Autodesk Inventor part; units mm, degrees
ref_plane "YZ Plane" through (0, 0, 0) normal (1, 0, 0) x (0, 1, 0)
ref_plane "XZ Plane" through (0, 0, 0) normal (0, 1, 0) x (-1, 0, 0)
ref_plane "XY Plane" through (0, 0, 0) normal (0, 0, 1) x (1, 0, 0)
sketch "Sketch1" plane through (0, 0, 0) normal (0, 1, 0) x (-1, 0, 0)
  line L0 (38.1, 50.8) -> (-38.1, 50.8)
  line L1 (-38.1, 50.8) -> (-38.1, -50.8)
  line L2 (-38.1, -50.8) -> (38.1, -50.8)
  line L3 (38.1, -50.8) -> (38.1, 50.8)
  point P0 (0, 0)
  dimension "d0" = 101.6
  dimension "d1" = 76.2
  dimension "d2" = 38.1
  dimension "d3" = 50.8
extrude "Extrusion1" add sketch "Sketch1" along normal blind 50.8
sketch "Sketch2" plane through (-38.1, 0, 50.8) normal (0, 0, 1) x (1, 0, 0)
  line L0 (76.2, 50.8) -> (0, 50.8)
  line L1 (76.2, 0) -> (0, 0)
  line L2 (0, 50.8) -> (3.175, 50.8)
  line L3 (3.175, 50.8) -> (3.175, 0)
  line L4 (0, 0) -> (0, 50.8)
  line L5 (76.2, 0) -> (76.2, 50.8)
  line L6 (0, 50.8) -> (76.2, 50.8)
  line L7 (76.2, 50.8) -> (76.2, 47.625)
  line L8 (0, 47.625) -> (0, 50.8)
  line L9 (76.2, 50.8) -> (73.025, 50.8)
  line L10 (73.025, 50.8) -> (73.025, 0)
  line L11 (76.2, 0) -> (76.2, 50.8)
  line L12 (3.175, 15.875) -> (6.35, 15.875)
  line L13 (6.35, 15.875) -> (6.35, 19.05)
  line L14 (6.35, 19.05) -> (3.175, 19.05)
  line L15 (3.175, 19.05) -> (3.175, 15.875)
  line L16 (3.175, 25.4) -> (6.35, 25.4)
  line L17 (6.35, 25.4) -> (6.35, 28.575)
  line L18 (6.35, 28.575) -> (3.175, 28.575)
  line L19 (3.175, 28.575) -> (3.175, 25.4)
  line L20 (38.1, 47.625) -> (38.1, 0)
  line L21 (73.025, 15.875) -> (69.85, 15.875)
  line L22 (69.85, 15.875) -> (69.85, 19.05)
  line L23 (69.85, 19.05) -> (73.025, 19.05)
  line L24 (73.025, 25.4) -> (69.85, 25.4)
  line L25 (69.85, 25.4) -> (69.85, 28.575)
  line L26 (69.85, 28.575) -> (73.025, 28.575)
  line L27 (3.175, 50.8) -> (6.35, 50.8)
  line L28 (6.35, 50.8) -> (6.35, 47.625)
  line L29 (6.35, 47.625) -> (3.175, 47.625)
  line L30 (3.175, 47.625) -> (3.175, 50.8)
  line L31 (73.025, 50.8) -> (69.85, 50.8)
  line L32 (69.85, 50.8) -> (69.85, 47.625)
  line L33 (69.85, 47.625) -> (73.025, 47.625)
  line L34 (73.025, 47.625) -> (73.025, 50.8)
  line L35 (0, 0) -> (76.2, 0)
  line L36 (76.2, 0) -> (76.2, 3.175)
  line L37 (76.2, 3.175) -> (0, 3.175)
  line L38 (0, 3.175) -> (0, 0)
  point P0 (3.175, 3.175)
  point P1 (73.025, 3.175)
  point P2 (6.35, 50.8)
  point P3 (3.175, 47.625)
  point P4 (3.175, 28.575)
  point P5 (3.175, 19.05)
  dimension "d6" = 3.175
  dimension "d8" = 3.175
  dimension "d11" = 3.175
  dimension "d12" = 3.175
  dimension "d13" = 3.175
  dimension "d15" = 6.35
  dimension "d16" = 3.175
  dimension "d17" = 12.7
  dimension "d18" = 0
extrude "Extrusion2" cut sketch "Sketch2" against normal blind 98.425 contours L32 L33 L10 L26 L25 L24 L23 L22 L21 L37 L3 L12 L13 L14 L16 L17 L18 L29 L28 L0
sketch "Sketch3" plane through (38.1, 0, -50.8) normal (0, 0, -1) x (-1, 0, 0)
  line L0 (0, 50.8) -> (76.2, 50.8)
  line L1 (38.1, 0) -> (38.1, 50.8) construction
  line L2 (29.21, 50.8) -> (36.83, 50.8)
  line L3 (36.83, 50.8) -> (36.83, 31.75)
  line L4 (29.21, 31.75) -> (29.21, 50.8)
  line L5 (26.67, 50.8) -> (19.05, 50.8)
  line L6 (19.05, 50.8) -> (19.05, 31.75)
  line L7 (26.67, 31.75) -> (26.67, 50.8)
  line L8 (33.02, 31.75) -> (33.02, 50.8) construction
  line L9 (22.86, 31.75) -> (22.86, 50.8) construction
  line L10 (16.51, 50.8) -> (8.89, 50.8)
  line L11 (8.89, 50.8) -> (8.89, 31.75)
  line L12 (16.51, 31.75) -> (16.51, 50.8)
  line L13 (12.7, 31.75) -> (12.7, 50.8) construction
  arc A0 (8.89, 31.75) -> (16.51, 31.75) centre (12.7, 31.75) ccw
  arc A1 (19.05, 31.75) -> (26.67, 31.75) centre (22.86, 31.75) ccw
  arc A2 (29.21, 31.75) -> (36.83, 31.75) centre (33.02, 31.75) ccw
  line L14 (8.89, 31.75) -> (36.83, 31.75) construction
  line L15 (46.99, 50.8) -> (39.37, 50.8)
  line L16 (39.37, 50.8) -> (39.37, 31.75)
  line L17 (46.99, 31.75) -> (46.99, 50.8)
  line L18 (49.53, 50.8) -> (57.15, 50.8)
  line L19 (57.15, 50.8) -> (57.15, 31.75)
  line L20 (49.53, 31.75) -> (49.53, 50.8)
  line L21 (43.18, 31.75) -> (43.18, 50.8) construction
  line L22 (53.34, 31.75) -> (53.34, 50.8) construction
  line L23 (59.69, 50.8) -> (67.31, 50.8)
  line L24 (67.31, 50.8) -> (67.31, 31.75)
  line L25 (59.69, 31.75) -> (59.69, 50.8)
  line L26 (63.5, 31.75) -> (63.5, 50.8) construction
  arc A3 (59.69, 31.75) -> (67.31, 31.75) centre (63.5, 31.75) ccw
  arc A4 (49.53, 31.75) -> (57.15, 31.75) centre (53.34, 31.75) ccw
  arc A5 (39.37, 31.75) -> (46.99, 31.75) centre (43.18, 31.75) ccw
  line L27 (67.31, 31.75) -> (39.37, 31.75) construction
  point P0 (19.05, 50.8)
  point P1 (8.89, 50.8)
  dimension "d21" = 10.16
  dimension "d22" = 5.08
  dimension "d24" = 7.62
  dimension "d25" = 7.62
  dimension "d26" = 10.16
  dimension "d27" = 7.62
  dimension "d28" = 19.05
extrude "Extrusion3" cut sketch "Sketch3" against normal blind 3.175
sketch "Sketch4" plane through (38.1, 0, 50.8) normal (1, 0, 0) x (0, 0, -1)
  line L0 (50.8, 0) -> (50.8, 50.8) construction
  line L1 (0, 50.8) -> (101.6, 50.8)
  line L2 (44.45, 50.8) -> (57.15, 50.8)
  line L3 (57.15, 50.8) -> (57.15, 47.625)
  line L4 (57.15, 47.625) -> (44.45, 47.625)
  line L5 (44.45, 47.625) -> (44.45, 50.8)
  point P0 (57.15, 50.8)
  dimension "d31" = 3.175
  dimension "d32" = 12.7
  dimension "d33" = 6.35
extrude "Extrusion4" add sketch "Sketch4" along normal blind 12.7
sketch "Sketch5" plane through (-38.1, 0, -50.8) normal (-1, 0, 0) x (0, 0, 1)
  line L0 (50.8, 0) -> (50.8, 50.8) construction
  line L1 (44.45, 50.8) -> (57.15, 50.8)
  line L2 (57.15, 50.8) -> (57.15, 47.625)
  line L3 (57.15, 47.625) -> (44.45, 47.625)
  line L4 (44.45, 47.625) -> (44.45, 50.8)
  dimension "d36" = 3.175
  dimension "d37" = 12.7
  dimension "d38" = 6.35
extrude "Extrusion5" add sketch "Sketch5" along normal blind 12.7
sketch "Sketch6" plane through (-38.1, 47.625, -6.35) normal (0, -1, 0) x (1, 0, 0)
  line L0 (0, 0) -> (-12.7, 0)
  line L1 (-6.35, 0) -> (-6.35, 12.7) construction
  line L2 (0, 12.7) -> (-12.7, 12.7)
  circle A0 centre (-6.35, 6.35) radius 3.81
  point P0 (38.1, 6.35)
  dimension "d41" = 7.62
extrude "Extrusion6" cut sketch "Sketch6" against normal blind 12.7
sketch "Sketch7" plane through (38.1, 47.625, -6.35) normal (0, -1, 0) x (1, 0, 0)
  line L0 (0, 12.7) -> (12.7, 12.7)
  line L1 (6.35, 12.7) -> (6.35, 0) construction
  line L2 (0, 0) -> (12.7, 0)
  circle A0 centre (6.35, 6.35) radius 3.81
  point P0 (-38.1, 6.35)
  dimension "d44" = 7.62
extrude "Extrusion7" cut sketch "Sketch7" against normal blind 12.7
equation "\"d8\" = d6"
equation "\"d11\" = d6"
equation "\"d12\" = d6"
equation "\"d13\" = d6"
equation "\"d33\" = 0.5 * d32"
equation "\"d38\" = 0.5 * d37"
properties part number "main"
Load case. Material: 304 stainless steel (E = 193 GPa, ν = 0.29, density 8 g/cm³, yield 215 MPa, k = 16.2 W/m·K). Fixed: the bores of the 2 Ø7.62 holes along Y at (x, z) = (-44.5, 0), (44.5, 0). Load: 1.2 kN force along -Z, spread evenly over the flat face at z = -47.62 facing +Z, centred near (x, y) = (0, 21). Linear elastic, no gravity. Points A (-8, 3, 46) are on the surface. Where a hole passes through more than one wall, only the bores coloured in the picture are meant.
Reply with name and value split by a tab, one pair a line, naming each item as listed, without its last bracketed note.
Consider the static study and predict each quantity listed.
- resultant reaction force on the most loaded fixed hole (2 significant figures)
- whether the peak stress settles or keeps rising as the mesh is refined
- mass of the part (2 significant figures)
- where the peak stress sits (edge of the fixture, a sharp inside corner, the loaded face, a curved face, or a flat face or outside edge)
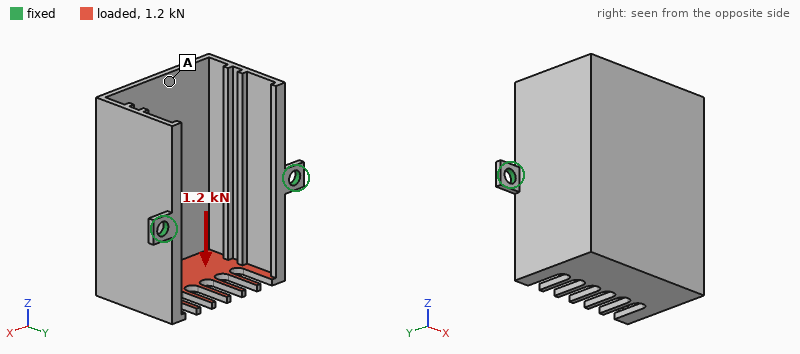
resultant reaction force on the most loaded fixed hole	600 N
whether the peak stress settles or keeps rising as the mesh is refined	keeps rising
mass of the part	550 g
where the peak stress sits	edge of the fixture
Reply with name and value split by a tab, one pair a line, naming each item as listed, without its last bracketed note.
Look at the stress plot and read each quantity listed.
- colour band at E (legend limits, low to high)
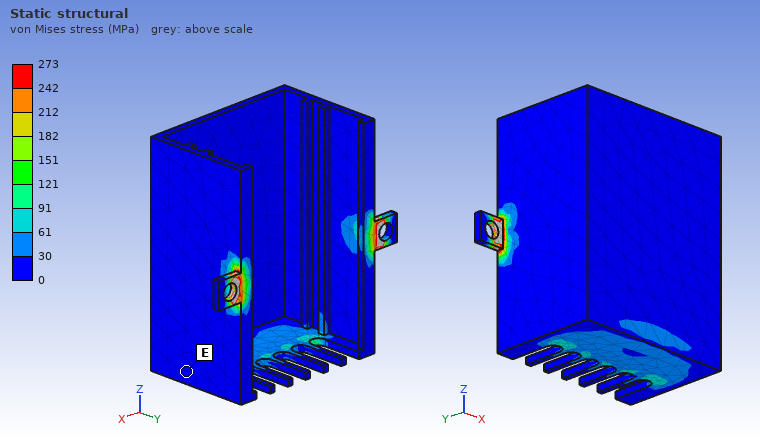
colour band at E	0 to 30 MPa
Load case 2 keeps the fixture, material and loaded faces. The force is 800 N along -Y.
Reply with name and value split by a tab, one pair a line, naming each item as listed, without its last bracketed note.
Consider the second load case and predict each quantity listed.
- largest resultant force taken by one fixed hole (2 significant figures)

largest resultant force taken by one fixed hole	400 N
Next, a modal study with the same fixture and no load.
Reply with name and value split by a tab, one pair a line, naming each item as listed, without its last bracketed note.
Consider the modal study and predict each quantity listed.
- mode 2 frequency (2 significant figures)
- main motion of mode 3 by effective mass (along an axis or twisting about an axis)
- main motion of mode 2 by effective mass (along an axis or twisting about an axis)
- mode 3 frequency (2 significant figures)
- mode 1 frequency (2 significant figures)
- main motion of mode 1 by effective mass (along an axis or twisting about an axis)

mode 2 frequency	570 Hz
main motion of mode 3 by effective mass	along X
main motion of mode 2 by effective mass	along X
mode 3 frequency	760 Hz
mode 1 frequency	380 Hz
main motion of mode 1 by effective mass	along Z
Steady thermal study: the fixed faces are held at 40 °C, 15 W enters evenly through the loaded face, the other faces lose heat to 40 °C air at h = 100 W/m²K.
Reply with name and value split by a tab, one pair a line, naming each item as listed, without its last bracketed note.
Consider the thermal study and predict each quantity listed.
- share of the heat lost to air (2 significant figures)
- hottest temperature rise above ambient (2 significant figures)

share of the heat lost to air	100 %
hottest temperature rise above ambient	30 K
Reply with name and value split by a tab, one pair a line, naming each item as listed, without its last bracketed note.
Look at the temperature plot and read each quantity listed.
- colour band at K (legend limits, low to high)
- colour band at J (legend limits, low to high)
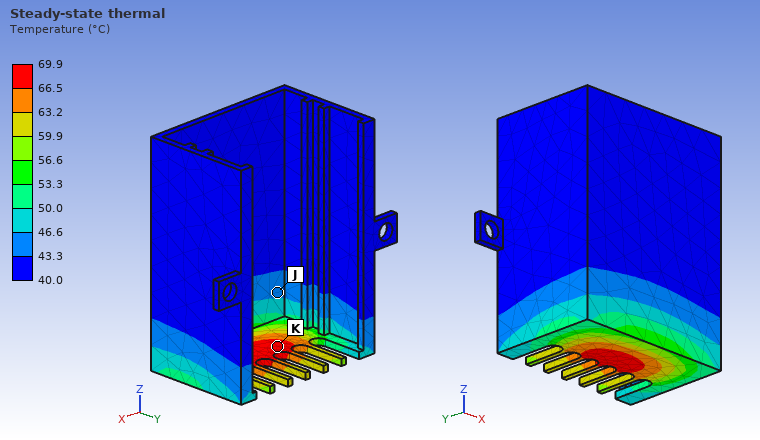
colour band at K	66.5 to 69.9 °C
colour band at J	43.3 to 46.6 °C
